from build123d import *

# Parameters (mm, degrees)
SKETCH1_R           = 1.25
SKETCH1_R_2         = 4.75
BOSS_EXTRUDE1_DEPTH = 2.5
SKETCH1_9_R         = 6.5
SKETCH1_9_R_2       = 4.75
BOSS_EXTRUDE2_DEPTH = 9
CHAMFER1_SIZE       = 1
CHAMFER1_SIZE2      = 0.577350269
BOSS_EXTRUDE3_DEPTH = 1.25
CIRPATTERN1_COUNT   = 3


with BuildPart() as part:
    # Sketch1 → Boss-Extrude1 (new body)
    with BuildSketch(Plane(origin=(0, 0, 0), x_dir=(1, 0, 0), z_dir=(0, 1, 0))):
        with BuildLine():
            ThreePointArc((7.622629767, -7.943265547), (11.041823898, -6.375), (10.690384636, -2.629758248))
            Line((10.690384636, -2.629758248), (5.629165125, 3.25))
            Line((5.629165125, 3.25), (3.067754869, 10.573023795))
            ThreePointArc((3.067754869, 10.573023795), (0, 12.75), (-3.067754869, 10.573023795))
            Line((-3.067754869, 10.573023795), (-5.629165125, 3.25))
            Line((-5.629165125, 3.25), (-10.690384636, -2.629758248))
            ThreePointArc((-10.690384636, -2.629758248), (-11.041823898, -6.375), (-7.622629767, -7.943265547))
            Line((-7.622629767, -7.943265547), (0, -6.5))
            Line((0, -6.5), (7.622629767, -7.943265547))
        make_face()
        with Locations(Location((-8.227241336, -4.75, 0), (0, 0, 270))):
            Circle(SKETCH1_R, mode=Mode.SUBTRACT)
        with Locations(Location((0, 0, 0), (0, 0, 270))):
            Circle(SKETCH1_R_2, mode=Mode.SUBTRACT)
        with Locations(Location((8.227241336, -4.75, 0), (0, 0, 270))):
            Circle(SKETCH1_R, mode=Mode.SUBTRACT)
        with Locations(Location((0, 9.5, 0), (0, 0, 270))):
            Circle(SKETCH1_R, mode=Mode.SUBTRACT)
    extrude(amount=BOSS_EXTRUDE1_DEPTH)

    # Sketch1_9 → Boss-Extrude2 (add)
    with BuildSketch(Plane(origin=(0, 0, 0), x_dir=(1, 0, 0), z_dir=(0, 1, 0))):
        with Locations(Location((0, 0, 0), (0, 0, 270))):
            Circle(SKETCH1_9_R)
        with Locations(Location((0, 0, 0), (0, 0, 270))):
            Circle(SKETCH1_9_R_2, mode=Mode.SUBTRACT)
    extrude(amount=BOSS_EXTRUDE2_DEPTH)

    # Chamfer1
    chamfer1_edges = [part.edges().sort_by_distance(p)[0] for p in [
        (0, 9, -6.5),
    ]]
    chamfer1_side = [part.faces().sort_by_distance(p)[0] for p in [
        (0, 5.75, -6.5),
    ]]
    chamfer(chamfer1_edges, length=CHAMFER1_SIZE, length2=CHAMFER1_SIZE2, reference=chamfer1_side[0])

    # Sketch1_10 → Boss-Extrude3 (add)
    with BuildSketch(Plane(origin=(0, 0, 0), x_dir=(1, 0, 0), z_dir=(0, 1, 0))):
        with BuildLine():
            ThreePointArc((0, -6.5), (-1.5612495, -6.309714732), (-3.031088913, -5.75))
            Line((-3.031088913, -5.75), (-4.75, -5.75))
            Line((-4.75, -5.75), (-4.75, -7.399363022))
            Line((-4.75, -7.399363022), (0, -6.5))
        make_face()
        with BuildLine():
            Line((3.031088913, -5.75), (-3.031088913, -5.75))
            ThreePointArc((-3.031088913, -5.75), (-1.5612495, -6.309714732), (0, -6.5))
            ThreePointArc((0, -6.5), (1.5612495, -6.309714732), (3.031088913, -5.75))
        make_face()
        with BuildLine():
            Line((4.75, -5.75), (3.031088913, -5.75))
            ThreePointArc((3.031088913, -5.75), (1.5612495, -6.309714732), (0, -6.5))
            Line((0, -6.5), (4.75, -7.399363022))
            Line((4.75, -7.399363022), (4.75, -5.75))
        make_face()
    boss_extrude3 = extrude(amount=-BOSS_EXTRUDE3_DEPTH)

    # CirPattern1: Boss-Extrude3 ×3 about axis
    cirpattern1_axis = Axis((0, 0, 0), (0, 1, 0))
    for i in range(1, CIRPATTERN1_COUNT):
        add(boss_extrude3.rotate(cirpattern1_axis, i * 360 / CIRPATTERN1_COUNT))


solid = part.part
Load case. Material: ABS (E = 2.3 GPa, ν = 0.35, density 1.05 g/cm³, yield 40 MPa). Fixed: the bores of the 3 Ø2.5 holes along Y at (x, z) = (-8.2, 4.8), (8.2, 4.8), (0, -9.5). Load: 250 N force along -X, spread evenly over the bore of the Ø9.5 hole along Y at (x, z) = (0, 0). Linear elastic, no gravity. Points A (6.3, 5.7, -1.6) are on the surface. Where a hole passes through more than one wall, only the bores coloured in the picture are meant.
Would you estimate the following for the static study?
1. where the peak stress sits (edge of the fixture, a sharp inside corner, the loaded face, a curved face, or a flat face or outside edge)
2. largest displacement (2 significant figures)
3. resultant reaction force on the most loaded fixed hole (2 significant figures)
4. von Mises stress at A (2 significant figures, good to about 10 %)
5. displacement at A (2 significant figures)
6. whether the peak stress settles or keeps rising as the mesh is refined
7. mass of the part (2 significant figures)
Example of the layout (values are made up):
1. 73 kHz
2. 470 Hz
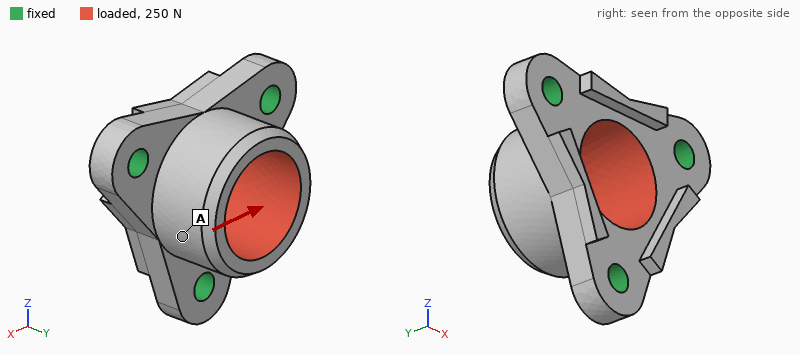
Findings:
1. edge of the fixture
2. 0.11 mm
3. 99 N
4. 4.2 MPa
5. 0.080 mm
6. keeps rising
7. 0.95 g
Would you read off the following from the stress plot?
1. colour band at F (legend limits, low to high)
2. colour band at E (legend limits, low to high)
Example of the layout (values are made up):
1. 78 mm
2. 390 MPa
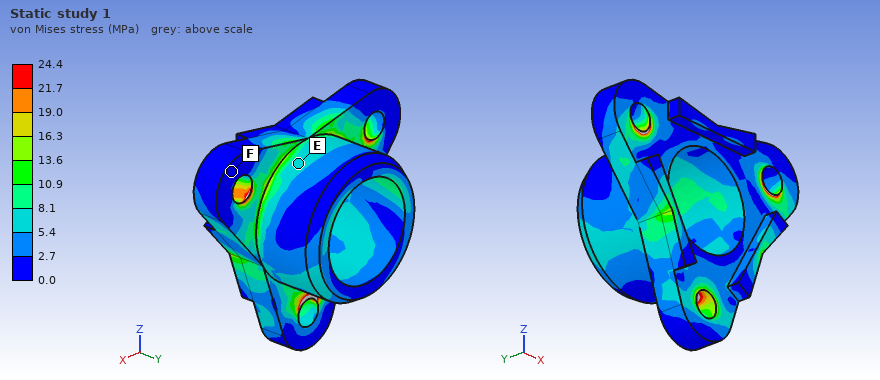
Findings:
1. 0.0 to 2.7 MPa
2. 5.4 to 8.1 MPa
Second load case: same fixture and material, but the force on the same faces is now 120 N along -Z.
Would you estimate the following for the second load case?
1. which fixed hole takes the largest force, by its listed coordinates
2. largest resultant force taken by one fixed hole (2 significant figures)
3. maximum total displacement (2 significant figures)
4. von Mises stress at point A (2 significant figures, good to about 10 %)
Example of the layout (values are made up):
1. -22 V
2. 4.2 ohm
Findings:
1. (0, -9.5)
2. 50 N
3. 61 µm
4. 2.7 MPa
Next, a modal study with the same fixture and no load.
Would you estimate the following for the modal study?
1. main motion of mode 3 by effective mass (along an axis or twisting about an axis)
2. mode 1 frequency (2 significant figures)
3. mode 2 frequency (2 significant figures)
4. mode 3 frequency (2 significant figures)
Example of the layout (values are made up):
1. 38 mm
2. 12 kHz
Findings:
1. along Y
2. 11 kHz
3. 11 kHz
4. 14 kHz
